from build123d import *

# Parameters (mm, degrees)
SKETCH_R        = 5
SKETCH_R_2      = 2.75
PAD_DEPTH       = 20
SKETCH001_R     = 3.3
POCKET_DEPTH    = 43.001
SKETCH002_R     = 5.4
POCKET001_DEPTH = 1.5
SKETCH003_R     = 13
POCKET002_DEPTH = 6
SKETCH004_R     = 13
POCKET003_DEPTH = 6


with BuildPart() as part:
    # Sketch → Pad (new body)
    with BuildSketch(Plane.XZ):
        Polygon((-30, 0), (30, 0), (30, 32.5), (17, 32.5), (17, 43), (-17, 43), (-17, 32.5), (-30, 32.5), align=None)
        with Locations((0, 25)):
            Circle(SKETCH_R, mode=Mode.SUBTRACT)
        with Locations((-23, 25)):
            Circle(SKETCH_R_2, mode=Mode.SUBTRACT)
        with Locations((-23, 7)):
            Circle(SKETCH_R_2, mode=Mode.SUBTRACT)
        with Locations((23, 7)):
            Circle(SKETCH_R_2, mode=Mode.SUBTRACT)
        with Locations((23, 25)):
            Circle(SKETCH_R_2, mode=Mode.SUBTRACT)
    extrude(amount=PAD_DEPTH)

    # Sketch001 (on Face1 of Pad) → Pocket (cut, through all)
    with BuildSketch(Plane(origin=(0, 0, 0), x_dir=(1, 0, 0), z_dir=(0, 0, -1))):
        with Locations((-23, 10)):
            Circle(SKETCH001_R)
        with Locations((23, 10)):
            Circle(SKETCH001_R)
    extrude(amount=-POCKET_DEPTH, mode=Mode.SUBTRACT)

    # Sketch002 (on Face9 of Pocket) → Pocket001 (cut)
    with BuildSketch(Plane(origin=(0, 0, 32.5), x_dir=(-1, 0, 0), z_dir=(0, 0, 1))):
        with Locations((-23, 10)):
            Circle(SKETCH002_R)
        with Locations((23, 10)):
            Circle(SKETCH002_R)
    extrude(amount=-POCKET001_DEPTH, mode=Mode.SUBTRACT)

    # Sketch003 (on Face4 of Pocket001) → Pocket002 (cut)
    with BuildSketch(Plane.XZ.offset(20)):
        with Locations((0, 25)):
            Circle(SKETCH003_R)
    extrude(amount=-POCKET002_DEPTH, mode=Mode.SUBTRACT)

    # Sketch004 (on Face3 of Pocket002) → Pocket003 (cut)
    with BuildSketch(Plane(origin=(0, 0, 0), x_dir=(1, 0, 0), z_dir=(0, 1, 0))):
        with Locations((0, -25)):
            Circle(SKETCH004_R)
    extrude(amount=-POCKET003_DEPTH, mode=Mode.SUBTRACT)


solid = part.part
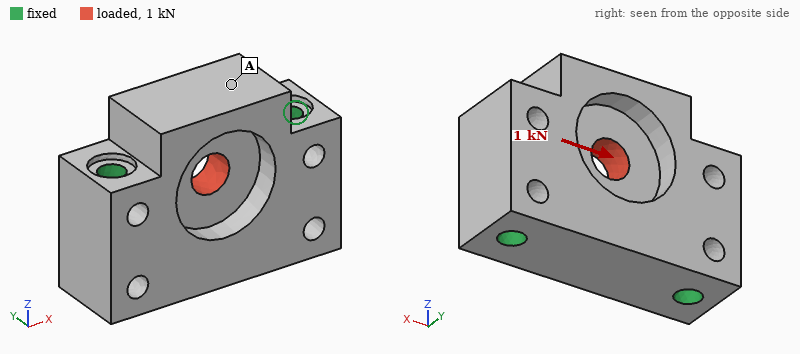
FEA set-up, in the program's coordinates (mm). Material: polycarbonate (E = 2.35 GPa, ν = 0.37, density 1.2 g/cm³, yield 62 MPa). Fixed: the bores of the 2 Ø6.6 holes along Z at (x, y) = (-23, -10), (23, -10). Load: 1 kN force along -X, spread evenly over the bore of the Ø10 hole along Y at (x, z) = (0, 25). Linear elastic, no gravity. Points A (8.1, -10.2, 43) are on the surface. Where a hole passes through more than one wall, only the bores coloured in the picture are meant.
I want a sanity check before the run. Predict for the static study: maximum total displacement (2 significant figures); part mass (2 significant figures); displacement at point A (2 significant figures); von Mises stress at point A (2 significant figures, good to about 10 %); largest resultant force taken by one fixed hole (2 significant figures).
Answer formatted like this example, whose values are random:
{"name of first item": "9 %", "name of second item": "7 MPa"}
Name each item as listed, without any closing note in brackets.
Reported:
{"maximum total displacement": "28 µm", "part mass": "42 g", "displacement at point A": "13 µm", "von Mises stress at point A": "0.79 MPa", "largest resultant force taken by one fixed hole": "510 N"}
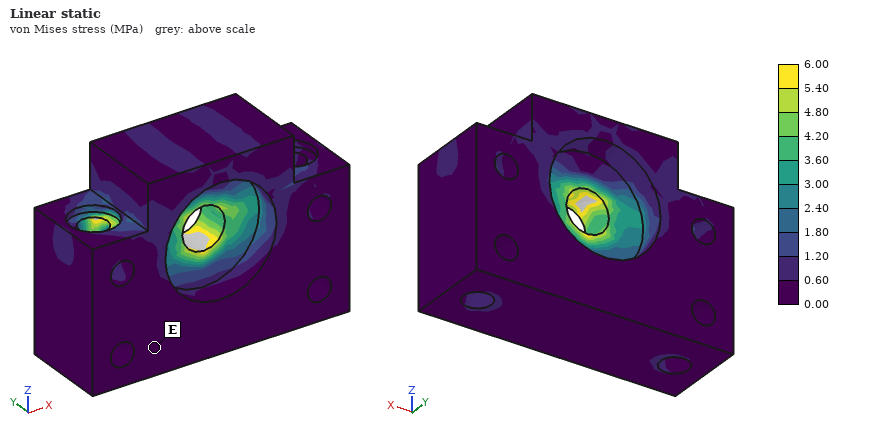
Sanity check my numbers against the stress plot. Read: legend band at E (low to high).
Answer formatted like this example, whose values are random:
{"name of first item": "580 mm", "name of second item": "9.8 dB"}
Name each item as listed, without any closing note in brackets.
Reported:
{"legend band at E": "0.00 to 0.60 MPa"}
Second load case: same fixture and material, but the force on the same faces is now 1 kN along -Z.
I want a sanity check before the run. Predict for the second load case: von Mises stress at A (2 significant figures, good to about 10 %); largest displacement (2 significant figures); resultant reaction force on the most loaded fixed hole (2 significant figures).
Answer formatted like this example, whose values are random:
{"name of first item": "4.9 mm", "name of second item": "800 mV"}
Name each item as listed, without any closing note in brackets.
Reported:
{"von Mises stress at A": "1.1 MPa", "largest displacement": "39 µm", "resultant reaction force on the most loaded fixed hole": "510 N"}
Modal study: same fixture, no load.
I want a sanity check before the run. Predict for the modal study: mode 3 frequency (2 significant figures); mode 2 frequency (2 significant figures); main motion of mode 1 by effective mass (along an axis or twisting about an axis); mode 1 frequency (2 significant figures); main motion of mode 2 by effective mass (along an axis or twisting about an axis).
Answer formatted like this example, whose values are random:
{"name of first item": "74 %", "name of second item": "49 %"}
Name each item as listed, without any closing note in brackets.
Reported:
{"mode 3 frequency": "7400 Hz", "mode 2 frequency": "6800 Hz", "main motion of mode 1 by effective mass": "along Y", "mode 1 frequency": "4200 Hz", "main motion of mode 2 by effective mass": "along Y"}
